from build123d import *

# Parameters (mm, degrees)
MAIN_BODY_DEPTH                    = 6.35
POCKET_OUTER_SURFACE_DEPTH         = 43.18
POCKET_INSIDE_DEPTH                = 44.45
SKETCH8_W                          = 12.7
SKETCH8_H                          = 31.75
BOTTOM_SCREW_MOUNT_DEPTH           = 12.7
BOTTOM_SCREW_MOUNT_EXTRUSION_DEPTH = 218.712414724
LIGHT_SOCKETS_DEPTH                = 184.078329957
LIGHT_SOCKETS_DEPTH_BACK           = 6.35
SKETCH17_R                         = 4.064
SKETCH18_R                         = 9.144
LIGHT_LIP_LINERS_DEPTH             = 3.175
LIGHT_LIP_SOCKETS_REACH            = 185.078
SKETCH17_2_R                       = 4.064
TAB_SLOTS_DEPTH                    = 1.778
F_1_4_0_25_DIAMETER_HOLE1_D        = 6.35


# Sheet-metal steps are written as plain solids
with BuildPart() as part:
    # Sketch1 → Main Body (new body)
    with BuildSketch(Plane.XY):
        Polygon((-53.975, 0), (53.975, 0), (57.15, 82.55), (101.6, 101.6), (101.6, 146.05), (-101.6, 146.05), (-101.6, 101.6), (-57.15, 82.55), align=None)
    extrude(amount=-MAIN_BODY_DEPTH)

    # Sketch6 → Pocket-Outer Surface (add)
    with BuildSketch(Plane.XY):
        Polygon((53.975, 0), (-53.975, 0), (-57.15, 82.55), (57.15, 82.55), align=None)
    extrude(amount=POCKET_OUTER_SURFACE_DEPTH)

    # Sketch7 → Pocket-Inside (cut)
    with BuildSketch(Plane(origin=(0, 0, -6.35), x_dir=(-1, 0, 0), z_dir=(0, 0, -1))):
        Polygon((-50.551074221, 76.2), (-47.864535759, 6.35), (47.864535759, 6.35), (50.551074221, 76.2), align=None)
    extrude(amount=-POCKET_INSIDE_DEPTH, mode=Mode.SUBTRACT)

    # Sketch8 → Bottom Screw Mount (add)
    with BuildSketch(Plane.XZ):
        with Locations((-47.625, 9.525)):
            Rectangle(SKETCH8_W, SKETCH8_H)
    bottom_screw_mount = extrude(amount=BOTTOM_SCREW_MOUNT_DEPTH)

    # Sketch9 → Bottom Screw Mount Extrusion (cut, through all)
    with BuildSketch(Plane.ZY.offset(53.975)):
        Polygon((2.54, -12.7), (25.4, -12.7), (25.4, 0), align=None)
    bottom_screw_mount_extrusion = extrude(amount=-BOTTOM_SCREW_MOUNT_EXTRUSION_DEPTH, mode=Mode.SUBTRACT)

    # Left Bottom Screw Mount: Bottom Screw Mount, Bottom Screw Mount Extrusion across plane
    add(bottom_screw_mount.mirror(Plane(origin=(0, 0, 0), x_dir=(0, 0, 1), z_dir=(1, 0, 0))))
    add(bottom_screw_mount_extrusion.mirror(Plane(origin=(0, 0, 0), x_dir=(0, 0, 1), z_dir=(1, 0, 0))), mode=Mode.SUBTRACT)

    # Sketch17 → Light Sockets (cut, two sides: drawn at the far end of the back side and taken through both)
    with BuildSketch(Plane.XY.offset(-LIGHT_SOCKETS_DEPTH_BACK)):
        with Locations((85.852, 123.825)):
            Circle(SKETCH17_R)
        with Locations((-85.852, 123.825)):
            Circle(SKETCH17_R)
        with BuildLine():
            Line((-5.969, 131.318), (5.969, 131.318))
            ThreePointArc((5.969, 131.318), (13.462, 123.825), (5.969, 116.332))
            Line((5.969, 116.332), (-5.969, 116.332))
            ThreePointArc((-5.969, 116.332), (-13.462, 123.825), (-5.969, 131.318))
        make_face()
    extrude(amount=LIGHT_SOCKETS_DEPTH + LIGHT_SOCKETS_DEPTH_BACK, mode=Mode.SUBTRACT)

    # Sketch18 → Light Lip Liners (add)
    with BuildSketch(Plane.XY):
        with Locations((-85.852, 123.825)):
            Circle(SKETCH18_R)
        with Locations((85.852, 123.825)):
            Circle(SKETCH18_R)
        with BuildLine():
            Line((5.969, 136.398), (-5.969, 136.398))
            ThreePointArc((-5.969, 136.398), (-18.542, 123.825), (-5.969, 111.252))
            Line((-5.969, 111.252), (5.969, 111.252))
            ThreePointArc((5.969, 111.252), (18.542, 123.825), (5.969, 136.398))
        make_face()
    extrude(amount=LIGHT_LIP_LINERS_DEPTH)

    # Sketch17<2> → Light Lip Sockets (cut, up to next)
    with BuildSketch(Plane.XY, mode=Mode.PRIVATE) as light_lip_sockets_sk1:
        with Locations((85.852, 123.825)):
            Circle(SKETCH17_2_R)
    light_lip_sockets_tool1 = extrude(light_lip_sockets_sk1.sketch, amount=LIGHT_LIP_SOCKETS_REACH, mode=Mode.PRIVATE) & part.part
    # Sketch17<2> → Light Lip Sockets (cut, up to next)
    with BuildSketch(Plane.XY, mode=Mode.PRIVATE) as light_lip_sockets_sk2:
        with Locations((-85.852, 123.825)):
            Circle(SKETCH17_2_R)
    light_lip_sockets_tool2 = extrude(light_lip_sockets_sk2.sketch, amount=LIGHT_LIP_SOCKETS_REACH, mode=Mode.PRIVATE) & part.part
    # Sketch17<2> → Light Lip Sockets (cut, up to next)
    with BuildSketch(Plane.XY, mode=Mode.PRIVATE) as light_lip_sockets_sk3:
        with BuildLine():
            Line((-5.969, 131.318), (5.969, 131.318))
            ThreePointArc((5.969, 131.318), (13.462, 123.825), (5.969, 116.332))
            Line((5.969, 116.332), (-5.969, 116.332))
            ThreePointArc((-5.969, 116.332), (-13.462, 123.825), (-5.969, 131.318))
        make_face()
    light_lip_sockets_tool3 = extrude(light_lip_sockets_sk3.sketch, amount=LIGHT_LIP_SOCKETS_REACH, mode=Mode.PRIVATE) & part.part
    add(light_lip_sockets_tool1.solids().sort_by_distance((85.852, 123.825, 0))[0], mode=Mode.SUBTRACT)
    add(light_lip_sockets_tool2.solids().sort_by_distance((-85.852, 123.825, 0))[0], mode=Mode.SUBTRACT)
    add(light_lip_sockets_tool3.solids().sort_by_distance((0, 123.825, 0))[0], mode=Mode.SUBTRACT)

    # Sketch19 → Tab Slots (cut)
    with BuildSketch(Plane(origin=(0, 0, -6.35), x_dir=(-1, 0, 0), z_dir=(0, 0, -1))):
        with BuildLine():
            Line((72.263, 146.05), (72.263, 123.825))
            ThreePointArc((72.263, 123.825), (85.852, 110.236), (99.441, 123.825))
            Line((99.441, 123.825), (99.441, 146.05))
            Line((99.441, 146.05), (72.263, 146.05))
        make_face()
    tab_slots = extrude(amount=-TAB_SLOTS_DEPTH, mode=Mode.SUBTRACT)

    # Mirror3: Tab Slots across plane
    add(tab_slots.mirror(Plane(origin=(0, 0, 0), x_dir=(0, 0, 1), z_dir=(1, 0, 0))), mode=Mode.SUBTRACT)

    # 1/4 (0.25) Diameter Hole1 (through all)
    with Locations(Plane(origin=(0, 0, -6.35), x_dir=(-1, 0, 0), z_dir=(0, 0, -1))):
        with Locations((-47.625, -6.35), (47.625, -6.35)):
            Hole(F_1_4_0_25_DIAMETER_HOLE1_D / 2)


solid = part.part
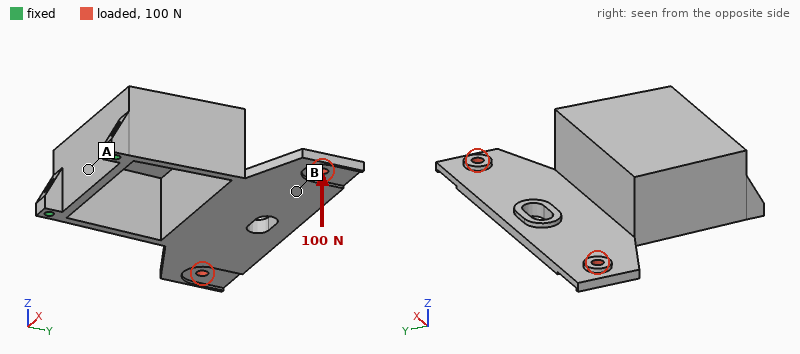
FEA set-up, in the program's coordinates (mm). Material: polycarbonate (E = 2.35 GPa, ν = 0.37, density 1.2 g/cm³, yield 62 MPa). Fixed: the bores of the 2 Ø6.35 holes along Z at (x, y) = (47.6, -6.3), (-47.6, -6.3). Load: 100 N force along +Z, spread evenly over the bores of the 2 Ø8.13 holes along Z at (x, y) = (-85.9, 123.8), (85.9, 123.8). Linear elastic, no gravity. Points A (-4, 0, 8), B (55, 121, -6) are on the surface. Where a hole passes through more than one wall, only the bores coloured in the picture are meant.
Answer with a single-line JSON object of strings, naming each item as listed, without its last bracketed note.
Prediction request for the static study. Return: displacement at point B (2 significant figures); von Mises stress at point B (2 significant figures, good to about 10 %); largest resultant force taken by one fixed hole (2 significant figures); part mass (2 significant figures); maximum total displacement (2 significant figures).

{"displacement at point B": "1.2 mm", "von Mises stress at point B": "3.0 MPa", "largest resultant force taken by one fixed hole": "53 N", "part mass": "270 g", "maximum total displacement": "2.8 mm"}
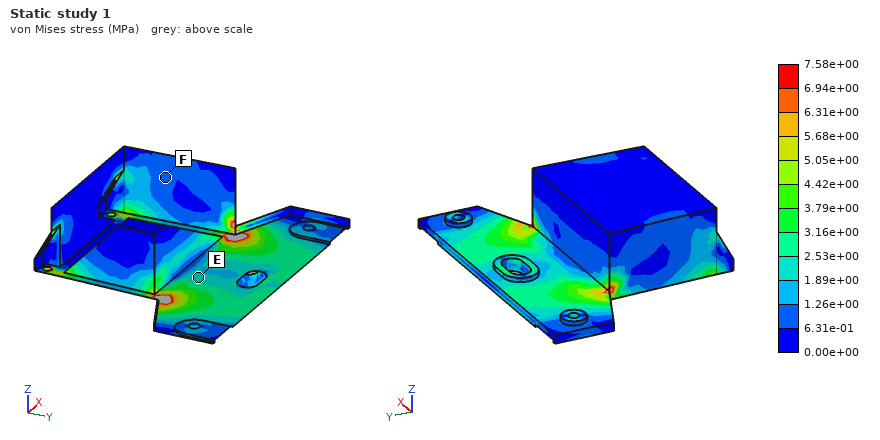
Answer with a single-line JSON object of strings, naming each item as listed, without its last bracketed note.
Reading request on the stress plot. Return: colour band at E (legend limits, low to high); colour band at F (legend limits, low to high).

{"colour band at E": "1.89e+00 to 2.53e+00 MPa", "colour band at F": "6.31e-01 to 1.26e+00 MPa"}
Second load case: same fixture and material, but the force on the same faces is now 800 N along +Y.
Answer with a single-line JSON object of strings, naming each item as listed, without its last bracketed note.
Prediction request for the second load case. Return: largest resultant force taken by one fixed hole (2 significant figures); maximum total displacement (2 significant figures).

{"largest resultant force taken by one fixed hole": "400 N", "maximum total displacement": "0.54 mm"}
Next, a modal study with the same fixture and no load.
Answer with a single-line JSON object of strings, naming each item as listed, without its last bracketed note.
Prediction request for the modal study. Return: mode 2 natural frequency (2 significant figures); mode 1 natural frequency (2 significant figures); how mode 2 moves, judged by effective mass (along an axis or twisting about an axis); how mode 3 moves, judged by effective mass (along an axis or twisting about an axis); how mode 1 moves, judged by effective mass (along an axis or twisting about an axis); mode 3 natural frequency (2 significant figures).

{"mode 2 natural frequency": "180 Hz", "mode 1 natural frequency": "170 Hz", "how mode 2 moves, judged by effective mass": "along X", "how mode 3 moves, judged by effective mass": "along X", "how mode 1 moves, judged by effective mass": "along Z", "mode 3 natural frequency": "320 Hz"}
